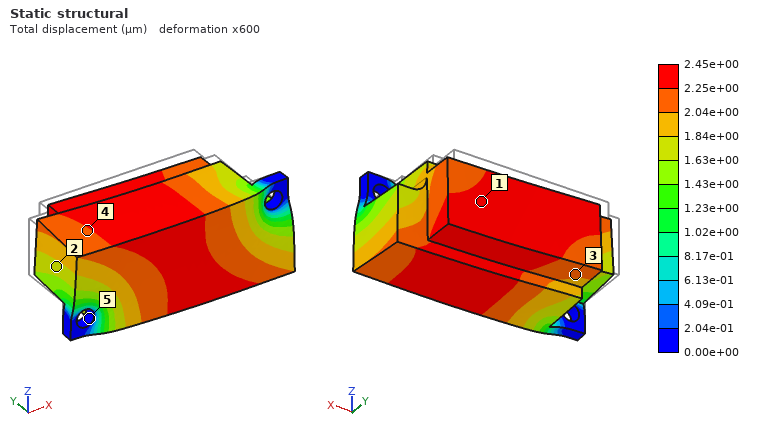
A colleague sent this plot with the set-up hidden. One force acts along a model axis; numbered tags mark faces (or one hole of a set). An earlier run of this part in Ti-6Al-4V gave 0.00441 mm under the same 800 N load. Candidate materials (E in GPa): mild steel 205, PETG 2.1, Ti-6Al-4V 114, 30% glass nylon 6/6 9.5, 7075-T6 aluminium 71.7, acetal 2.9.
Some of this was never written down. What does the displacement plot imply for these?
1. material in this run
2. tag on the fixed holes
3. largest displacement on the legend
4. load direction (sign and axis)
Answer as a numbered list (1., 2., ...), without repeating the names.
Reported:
1. mild steel
2. 5
3. 2.45e+00 µm
4. -Y
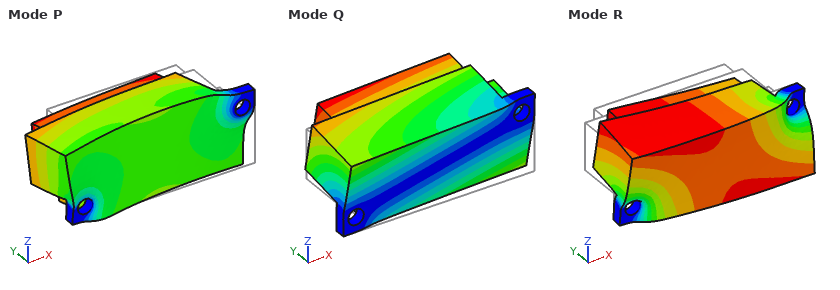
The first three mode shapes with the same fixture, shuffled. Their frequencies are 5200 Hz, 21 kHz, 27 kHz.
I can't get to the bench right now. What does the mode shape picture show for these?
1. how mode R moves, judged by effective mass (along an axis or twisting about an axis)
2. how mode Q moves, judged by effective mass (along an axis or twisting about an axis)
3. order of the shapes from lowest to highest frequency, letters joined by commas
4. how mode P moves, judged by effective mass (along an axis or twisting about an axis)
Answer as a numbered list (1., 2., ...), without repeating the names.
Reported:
1. along Y
2. along Z
3. Q, R, P
4. along X
